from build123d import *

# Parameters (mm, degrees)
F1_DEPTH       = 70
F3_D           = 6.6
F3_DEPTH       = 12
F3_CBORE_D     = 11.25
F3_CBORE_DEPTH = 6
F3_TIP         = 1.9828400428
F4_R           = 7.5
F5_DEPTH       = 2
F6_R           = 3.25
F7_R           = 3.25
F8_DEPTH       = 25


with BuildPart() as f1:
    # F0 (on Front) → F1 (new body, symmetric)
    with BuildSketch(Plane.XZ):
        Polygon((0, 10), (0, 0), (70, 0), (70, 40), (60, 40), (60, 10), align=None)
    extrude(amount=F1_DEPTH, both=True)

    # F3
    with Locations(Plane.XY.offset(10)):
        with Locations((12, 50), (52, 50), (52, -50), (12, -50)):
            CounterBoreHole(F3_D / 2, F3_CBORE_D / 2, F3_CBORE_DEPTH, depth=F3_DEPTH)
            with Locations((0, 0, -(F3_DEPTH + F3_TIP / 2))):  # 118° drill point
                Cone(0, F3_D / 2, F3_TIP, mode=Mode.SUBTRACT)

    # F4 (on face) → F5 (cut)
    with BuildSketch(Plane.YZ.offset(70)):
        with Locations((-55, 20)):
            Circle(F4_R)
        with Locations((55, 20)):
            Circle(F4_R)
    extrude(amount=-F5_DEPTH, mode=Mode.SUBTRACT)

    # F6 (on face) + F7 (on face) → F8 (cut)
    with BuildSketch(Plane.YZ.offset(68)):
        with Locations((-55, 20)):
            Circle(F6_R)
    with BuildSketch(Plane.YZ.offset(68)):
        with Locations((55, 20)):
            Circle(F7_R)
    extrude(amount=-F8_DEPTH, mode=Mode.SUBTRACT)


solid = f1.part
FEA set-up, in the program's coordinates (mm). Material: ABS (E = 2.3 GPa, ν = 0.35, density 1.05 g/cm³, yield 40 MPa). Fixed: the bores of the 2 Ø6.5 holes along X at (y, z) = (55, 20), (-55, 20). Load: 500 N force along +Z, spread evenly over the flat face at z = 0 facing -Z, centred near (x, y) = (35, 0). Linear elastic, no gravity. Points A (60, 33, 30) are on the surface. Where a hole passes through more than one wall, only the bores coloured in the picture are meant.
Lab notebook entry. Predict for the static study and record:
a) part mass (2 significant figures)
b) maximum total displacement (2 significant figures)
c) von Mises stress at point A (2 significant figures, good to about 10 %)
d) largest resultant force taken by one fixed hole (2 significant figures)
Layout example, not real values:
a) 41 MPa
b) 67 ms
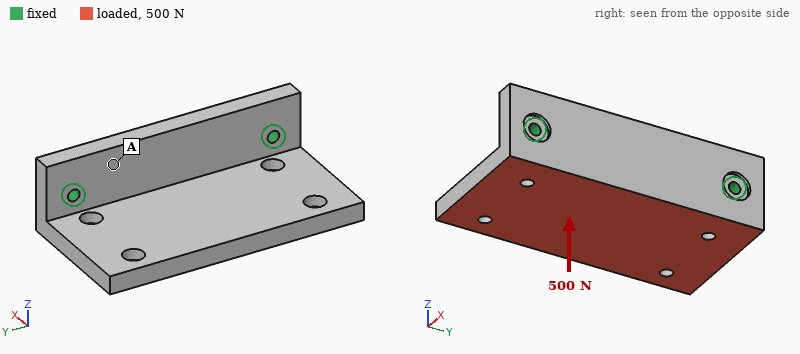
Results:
a) 140 g
b) 1.8 mm
c) 3.9 MPa
d) 250 N
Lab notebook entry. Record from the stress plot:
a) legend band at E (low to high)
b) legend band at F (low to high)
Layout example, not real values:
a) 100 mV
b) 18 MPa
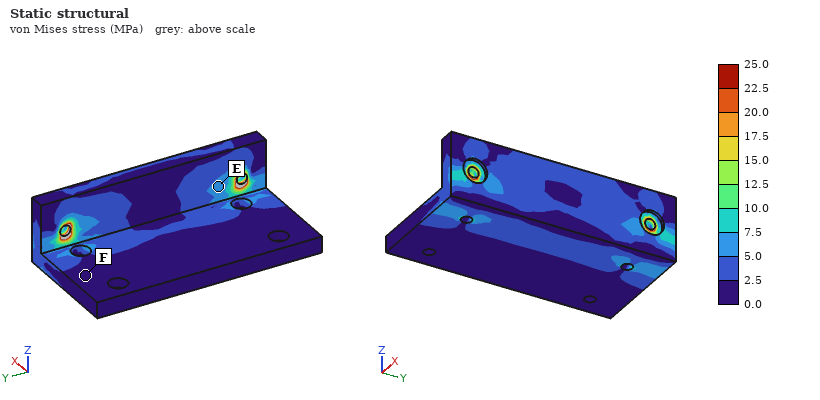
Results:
a) 5.0 to 7.5 MPa
b) 0.0 to 2.5 MPa
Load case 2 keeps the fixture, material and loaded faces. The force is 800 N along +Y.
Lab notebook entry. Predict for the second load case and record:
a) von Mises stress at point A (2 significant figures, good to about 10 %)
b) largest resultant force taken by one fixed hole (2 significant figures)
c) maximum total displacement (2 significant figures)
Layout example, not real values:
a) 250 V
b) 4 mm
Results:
a) 0.88 MPa
b) 470 N
c) 0.12 mm
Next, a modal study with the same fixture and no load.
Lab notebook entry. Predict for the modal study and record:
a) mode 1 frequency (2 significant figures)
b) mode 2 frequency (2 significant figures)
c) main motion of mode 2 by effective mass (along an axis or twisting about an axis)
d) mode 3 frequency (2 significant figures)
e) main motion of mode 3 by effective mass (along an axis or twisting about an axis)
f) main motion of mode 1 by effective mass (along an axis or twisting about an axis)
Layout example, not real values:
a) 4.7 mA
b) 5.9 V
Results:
a) 320 Hz
b) 660 Hz
c) twisting about X
d) 1200 Hz
e) along X
f) along Z
